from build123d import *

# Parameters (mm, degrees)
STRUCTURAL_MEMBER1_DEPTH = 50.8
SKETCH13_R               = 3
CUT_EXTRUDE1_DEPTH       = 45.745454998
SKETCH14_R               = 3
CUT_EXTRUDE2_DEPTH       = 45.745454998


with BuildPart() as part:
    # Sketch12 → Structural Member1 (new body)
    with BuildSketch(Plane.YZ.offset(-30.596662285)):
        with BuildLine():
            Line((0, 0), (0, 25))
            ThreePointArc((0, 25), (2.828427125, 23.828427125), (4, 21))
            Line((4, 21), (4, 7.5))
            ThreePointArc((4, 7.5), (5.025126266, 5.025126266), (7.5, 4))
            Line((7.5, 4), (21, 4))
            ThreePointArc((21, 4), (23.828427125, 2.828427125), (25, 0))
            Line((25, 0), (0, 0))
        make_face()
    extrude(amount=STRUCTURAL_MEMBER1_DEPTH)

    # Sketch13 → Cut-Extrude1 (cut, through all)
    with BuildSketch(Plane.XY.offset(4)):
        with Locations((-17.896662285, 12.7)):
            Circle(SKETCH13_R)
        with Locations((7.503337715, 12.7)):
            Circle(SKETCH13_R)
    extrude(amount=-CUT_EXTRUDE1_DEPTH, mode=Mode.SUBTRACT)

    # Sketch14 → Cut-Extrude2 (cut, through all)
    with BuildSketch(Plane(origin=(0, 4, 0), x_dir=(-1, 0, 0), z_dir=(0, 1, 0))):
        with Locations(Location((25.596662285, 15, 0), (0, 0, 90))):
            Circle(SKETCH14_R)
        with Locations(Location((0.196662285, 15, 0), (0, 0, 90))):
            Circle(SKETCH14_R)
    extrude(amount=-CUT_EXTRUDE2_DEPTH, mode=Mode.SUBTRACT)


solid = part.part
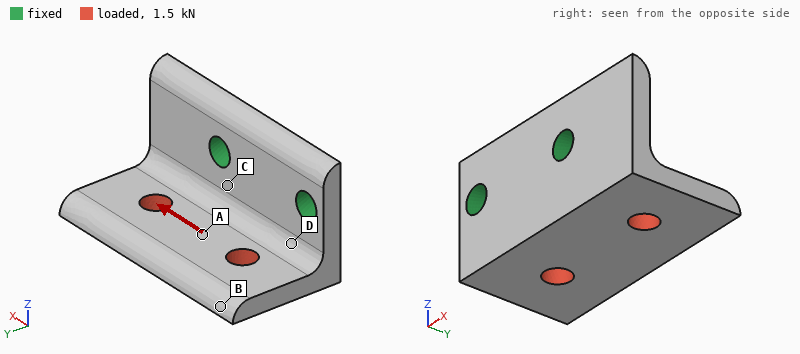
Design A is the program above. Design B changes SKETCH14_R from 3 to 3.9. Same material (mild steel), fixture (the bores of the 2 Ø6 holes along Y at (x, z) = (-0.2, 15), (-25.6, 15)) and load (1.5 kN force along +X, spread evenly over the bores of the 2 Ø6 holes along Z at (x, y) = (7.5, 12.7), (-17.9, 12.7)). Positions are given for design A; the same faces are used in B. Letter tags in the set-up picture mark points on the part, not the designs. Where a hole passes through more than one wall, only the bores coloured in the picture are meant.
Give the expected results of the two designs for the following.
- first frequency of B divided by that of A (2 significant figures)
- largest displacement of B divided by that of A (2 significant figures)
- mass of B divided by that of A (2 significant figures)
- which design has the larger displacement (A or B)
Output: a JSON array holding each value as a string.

["1.1", "0.84", "0.98", "A"]
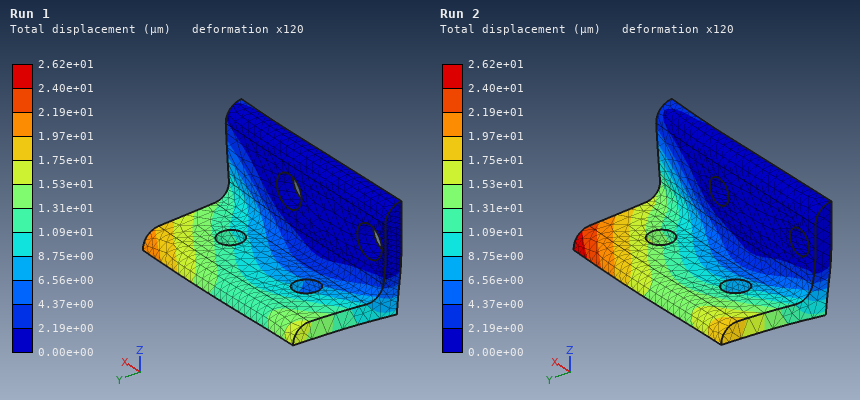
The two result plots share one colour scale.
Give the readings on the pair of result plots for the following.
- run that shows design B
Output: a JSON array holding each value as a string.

["Run 1"]
